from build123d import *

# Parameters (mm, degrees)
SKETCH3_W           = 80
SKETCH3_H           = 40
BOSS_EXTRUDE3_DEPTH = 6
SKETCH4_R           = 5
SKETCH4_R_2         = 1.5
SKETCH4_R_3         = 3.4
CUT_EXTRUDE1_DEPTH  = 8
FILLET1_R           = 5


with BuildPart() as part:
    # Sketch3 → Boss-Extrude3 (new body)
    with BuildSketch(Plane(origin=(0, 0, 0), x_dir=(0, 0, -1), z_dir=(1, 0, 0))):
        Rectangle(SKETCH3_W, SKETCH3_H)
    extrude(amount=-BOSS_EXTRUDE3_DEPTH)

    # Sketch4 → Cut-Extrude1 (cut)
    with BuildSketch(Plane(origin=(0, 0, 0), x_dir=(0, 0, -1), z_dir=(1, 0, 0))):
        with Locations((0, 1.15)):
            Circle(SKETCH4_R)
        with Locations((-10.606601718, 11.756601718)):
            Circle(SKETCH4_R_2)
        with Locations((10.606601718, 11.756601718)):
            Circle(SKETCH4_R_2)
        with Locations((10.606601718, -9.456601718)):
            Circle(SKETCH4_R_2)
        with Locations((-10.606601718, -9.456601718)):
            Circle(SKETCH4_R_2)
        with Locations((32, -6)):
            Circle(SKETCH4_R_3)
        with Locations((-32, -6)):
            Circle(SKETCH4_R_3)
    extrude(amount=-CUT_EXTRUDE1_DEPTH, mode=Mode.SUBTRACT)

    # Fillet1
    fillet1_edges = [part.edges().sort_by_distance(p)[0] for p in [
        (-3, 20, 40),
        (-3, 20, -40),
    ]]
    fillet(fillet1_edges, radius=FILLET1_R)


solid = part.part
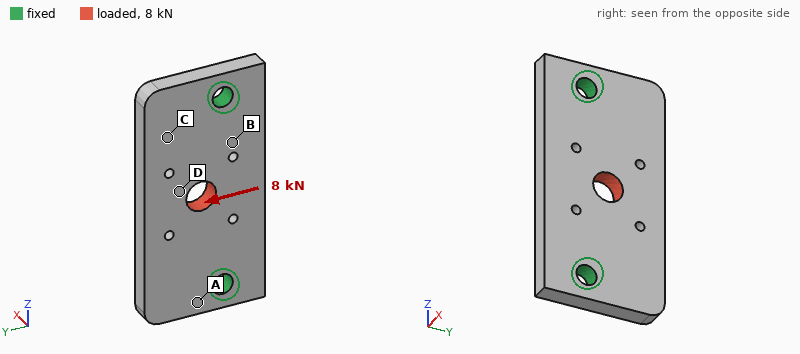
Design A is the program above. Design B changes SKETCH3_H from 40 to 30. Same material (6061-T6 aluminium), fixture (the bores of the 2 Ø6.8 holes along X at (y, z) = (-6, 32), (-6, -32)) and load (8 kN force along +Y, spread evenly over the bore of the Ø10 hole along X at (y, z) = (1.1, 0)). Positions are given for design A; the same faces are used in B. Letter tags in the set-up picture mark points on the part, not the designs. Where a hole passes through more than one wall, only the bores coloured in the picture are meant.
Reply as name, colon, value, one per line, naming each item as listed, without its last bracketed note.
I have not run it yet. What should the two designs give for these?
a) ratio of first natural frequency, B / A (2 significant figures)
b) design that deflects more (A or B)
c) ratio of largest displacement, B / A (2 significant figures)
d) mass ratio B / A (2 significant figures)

ratio of first natural frequency, B / A: 1.3
design that deflects more: B
ratio of largest displacement, B / A: 1.5
mass ratio B / A: 0.73
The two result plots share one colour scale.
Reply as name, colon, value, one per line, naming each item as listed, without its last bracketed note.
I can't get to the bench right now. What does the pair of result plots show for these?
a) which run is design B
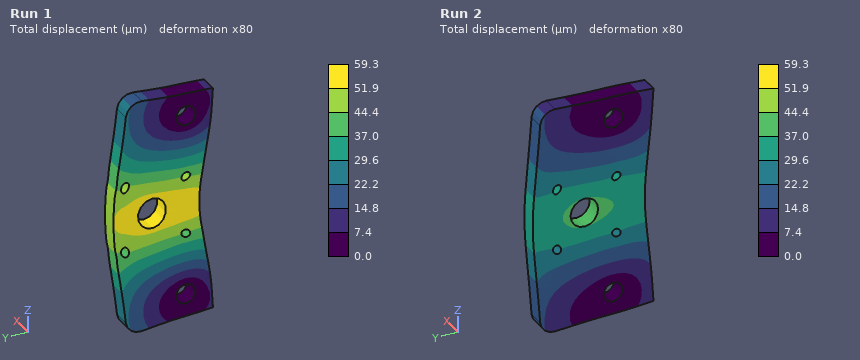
which run is design B: Run 1
